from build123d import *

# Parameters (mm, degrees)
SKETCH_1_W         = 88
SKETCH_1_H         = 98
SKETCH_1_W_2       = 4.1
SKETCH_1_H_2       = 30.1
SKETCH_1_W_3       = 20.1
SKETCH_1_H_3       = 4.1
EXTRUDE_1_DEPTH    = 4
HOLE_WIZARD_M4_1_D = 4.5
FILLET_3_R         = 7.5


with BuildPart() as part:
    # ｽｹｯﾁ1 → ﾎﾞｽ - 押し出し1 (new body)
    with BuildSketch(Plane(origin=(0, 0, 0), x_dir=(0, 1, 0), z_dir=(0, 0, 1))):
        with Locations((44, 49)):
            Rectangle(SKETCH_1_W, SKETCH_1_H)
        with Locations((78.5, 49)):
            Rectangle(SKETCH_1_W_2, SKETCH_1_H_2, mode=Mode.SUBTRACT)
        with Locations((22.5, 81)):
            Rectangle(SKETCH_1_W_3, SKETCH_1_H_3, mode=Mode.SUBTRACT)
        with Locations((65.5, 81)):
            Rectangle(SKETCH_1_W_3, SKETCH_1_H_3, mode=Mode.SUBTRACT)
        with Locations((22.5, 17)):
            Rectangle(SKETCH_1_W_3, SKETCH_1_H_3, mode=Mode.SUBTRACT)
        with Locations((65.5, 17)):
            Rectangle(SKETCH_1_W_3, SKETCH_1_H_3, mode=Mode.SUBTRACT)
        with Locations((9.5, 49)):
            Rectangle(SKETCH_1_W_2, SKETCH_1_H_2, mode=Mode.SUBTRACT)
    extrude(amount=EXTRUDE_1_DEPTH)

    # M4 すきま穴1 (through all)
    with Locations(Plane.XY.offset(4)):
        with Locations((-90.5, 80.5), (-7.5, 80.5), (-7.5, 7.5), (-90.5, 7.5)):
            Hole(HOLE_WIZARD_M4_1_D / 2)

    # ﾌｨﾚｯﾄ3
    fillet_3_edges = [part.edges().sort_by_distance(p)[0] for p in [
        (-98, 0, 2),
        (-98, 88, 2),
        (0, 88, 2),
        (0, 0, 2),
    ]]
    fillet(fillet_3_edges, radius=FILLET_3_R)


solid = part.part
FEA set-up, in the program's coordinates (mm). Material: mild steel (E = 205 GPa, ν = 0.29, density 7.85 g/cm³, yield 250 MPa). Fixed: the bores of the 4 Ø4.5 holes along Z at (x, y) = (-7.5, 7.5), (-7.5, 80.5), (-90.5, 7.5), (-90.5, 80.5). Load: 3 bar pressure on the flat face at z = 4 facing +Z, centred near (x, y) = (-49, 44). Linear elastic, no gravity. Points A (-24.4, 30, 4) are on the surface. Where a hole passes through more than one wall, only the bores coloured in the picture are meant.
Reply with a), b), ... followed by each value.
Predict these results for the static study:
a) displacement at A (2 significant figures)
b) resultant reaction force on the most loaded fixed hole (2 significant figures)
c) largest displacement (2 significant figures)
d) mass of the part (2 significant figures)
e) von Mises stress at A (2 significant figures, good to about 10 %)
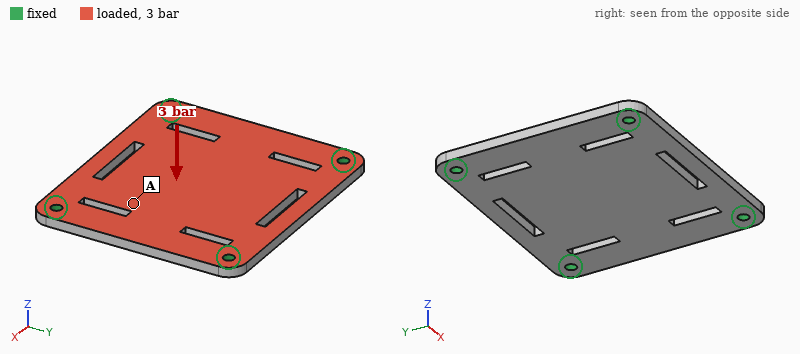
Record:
a) 50 µm
b) 600 N
c) 77 µm
d) 250 g
e) 23 MPa
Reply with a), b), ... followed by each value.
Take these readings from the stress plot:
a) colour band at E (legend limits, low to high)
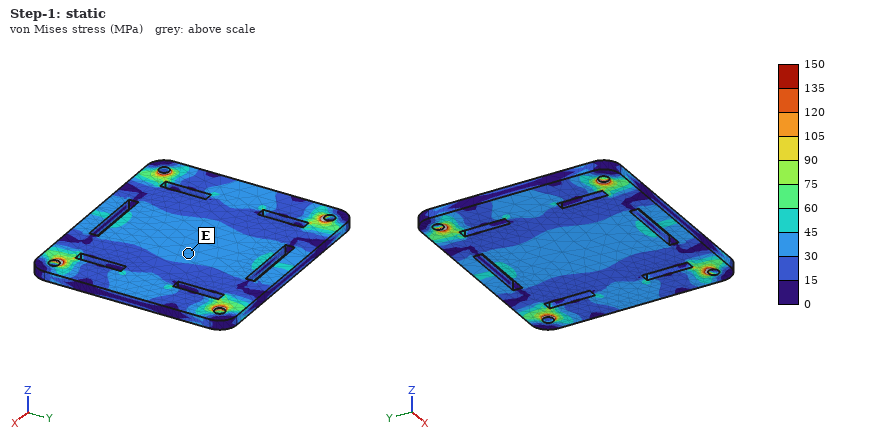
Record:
a) 30 to 45 MPa
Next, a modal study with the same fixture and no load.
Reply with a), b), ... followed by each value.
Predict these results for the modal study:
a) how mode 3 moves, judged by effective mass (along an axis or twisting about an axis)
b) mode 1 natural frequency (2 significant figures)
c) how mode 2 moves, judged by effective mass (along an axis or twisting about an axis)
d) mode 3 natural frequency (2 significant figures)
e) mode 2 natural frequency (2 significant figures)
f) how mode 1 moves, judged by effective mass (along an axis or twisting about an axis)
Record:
a) twisting about Y
b) 2100 Hz
c) twisting about X
d) 4000 Hz
e) 3400 Hz
f) along Z
